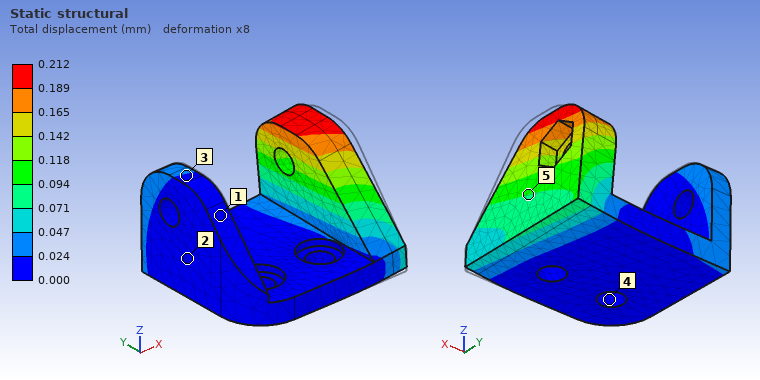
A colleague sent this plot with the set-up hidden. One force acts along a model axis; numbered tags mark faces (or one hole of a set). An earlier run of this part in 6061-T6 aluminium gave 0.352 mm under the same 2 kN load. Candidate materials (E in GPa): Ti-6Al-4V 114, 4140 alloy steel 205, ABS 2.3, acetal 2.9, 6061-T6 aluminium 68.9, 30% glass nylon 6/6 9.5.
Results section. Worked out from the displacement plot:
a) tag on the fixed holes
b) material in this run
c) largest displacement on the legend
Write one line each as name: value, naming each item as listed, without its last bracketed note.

tag on the fixed holes: 4
material in this run: Ti-6Al-4V
largest displacement on the legend: 0.212 mm
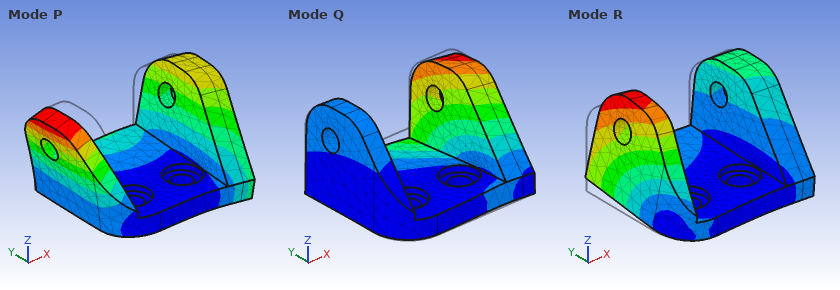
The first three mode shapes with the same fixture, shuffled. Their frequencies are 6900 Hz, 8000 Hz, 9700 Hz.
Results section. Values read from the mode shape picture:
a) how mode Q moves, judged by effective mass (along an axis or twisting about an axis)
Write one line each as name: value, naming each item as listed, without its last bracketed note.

how mode Q moves, judged by effective mass: along Z
